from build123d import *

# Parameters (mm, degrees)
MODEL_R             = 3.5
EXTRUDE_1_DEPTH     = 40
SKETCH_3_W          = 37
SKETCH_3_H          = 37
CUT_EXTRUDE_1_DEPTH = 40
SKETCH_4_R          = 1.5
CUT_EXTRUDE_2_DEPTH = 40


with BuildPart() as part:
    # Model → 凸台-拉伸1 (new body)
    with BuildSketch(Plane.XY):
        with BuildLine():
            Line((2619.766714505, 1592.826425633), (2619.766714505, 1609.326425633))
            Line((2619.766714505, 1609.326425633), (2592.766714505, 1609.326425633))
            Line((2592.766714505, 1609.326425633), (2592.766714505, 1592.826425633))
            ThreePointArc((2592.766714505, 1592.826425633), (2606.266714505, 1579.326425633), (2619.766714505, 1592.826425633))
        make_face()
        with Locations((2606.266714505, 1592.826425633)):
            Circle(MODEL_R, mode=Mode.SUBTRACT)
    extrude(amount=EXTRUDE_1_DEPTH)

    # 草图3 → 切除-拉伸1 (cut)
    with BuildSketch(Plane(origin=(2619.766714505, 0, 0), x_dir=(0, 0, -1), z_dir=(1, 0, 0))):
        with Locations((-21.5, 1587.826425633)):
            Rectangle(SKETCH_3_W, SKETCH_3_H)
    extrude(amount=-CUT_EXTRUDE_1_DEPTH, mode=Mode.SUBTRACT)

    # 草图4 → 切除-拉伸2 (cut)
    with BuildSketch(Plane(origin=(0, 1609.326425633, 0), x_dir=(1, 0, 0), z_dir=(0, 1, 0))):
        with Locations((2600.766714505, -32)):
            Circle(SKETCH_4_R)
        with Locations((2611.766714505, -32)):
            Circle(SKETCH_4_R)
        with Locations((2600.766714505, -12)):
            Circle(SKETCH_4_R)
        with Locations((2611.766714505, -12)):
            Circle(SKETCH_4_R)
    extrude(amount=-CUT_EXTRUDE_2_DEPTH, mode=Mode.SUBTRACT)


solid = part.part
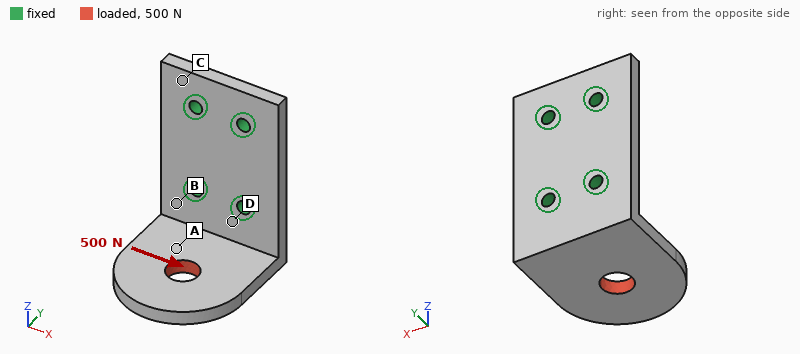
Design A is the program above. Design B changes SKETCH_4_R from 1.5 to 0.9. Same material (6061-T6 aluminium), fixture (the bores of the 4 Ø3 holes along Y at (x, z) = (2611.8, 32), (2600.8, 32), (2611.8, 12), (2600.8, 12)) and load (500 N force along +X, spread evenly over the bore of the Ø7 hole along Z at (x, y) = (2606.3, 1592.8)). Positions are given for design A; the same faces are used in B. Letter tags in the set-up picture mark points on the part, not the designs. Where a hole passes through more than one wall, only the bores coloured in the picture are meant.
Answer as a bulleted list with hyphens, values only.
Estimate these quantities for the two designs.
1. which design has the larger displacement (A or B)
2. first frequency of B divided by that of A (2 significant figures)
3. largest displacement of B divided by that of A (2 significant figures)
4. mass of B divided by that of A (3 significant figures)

- B
- 0.96
- 1.2
- 1.01
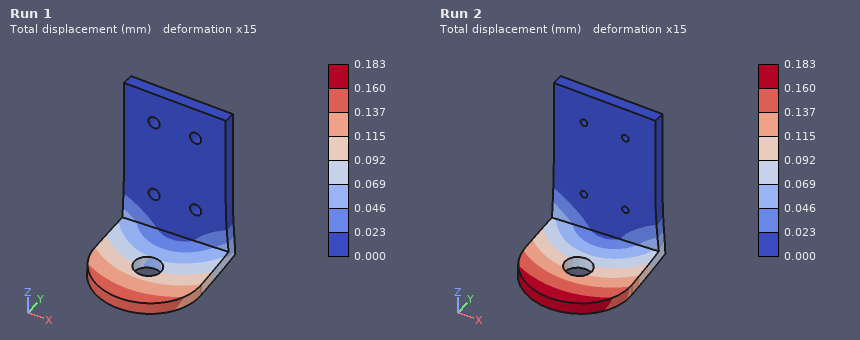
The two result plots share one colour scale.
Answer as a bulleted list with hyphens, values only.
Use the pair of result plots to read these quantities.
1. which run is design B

- Run 2
